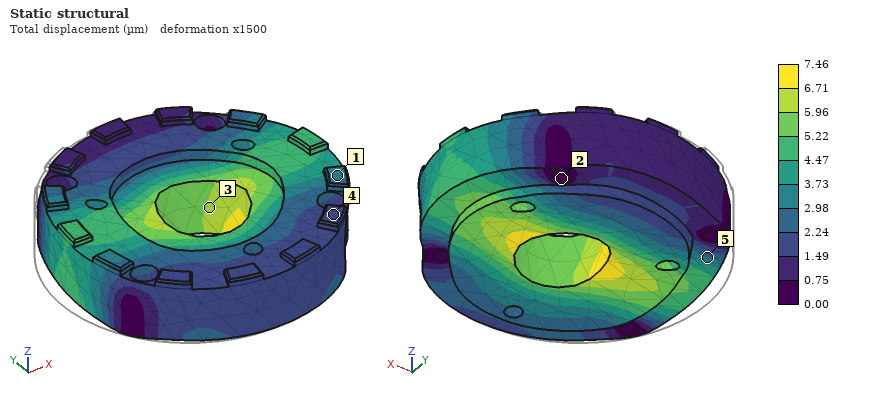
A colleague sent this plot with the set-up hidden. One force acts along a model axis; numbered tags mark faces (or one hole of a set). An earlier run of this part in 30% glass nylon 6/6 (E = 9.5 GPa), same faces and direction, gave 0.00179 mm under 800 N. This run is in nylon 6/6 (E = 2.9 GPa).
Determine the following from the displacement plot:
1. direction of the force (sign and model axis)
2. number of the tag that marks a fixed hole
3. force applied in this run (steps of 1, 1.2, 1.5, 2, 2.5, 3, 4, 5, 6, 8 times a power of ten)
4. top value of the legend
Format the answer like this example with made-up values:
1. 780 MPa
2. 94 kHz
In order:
1. +X
2. 2
3. 1 kN
4. 7.46 µm
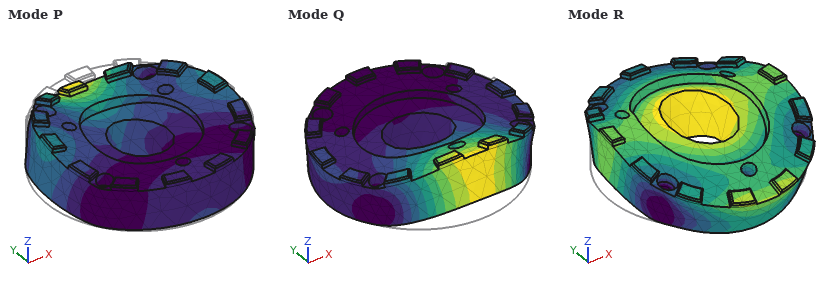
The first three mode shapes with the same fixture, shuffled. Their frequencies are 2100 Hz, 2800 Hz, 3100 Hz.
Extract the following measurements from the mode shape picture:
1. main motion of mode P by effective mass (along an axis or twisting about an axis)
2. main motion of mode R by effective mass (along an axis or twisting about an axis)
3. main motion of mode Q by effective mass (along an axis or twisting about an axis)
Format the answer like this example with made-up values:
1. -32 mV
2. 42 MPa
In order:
1. twisting about X
2. along Z
3. along Z
